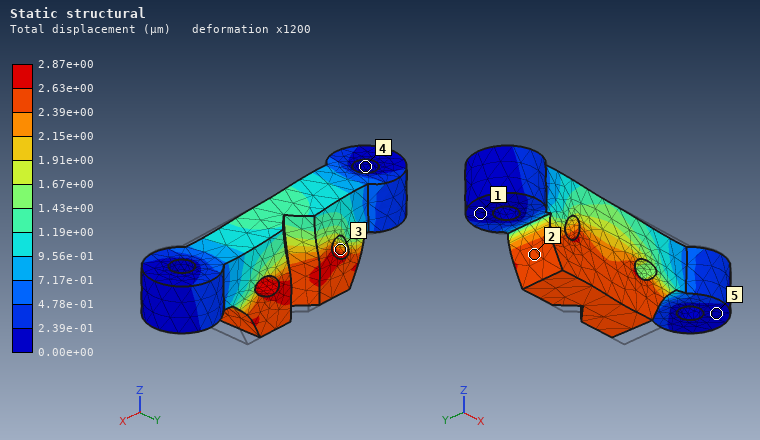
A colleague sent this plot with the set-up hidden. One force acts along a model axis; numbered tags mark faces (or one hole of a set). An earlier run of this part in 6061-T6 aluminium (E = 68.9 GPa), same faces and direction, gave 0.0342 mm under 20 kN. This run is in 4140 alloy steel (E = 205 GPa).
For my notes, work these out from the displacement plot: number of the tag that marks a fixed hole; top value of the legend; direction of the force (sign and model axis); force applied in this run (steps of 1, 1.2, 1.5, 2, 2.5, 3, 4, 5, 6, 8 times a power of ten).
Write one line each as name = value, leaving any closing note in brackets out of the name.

number of the tag that marks a fixed hole = 4
top value of the legend = 2.87e+00 µm
direction of the force = -X
force applied in this run = 5 kN
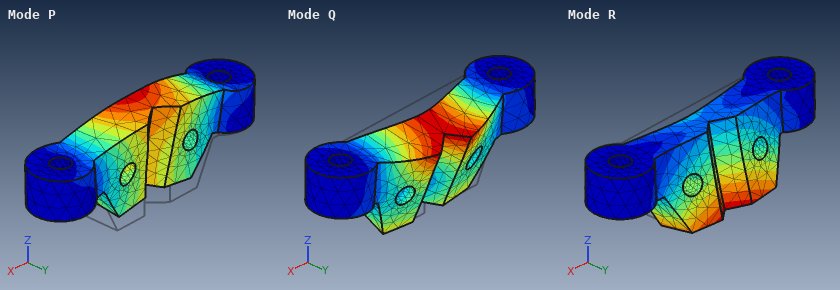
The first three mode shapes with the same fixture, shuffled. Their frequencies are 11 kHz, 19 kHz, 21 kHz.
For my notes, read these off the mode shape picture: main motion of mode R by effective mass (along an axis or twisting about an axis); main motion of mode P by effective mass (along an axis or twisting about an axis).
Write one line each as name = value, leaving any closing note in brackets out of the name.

main motion of mode R by effective mass = along Y
main motion of mode P by effective mass = along Z
